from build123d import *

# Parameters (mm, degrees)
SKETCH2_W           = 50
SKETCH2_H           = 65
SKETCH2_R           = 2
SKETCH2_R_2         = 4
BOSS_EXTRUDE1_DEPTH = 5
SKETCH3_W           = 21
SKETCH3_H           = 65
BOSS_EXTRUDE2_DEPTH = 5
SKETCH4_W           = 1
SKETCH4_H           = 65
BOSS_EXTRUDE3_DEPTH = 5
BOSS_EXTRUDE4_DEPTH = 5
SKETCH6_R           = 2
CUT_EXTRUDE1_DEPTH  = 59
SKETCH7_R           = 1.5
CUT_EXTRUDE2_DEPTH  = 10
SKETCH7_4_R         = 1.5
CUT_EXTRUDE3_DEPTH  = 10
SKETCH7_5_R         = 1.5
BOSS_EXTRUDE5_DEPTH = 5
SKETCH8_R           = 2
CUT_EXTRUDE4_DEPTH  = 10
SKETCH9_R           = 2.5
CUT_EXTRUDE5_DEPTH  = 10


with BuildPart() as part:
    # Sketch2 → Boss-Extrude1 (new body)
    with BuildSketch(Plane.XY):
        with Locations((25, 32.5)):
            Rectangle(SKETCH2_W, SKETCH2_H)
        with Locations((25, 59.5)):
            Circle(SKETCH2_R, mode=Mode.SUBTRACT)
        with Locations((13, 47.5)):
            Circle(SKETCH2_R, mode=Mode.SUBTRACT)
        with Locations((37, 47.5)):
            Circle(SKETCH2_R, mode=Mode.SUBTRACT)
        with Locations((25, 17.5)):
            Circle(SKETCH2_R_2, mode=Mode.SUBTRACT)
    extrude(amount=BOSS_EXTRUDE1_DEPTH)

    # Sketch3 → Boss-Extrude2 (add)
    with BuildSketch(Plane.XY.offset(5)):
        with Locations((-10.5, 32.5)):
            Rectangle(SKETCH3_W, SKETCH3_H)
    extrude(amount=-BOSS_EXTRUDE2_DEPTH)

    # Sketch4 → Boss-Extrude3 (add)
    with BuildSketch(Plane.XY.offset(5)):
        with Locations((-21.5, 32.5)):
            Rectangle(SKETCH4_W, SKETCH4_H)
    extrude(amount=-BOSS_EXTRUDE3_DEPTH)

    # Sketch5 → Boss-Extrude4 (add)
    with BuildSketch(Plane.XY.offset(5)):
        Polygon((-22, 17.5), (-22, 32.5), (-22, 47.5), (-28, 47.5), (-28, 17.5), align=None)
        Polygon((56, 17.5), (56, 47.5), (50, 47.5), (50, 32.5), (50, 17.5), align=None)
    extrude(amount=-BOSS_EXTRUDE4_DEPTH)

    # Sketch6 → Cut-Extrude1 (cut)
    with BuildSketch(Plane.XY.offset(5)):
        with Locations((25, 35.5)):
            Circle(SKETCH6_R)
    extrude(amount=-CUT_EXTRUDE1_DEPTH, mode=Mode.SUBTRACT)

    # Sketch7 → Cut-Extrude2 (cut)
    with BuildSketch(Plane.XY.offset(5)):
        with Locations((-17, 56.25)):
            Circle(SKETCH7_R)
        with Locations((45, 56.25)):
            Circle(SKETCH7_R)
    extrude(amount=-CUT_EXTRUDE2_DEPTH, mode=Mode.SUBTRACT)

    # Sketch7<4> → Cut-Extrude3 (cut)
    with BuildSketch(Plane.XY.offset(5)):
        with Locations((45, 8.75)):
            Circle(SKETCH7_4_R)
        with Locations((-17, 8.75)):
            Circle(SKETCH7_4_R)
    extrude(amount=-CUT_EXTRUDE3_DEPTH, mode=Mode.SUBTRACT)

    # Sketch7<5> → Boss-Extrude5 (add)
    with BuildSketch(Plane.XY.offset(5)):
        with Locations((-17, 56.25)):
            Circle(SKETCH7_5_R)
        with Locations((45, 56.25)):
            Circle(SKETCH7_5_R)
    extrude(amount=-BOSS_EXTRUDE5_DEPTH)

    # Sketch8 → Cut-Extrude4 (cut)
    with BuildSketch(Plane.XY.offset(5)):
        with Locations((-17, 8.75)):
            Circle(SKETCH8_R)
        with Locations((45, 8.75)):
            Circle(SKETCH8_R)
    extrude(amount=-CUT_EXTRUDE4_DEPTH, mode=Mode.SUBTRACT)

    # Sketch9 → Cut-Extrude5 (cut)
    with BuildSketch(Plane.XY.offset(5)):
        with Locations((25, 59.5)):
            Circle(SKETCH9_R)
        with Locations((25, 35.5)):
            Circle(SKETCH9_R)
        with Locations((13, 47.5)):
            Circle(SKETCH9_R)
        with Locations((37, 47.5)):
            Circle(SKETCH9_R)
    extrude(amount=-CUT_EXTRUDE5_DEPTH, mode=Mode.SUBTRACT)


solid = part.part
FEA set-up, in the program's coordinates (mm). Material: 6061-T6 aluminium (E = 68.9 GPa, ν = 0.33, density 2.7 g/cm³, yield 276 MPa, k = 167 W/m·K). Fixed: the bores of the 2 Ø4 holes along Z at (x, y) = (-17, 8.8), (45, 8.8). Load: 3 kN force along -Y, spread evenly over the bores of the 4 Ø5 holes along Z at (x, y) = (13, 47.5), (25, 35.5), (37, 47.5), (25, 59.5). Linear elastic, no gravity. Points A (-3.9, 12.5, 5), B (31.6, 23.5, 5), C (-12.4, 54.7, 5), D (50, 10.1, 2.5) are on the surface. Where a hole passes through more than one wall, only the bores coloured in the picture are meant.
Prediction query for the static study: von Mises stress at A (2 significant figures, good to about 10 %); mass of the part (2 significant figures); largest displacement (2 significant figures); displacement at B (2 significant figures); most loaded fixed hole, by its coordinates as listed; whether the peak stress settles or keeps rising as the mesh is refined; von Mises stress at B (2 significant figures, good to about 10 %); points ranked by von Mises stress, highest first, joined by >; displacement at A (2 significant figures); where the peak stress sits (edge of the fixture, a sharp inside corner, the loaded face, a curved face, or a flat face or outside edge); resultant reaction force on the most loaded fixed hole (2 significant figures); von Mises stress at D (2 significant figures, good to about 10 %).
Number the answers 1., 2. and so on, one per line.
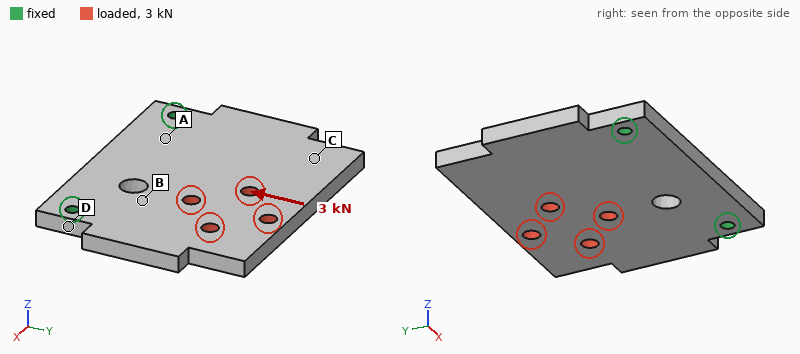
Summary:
1. 8.3 MPa
2. 66 g
3. 14 µm
4. 7.4 µm
5. (45, 8.8)
6. keeps rising
7. 15 MPa
8. D > B > A > C
9. 4.6 µm
10. edge of the fixture
11. 2.1 kN
12. 23 MPa
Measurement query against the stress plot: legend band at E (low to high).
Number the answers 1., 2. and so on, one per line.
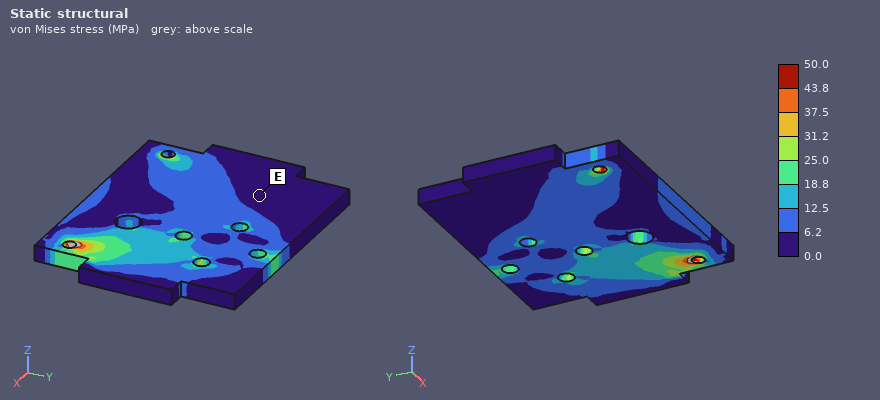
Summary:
1. 0.0 to 6.2 MPa
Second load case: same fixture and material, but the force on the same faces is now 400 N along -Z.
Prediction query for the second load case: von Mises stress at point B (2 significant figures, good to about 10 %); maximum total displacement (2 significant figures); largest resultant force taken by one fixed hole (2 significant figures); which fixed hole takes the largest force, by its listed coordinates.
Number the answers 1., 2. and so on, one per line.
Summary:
1. 32 MPa
2. 0.43 mm
3. 270 N
4. (45, 8.8)
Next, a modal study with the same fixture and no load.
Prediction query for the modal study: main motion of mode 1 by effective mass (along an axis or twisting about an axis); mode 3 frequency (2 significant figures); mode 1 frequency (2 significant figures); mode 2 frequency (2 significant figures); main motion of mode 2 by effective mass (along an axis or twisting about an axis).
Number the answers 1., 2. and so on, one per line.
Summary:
1. along Z
2. 5200 Hz
3. 1000 Hz
4. 2500 Hz
5. twisting about Y
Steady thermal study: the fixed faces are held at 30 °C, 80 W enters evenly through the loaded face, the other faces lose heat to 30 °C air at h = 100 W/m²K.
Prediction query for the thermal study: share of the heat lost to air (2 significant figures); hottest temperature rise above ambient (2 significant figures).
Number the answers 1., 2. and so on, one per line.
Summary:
1. 39 %
2. 59 K
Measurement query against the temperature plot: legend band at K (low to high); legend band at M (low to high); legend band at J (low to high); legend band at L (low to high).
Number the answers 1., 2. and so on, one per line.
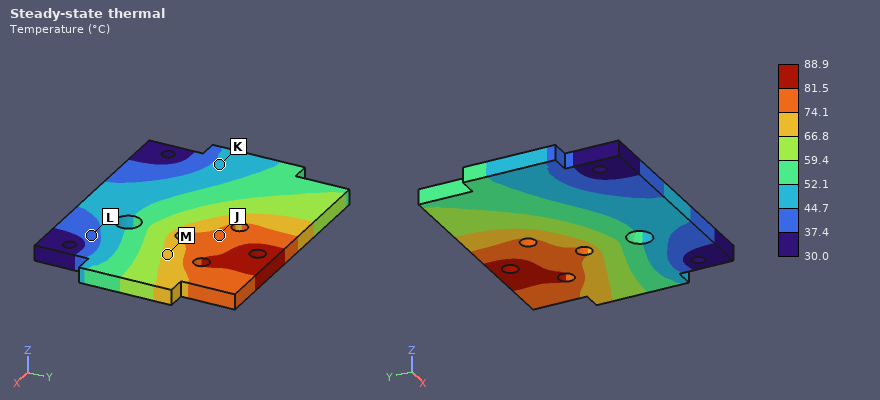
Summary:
1. 44.7 to 52.1 °C
2. 66.8 to 74.1 °C
3. 74.1 to 81.5 °C
4. 37.4 to 44.7 °C
